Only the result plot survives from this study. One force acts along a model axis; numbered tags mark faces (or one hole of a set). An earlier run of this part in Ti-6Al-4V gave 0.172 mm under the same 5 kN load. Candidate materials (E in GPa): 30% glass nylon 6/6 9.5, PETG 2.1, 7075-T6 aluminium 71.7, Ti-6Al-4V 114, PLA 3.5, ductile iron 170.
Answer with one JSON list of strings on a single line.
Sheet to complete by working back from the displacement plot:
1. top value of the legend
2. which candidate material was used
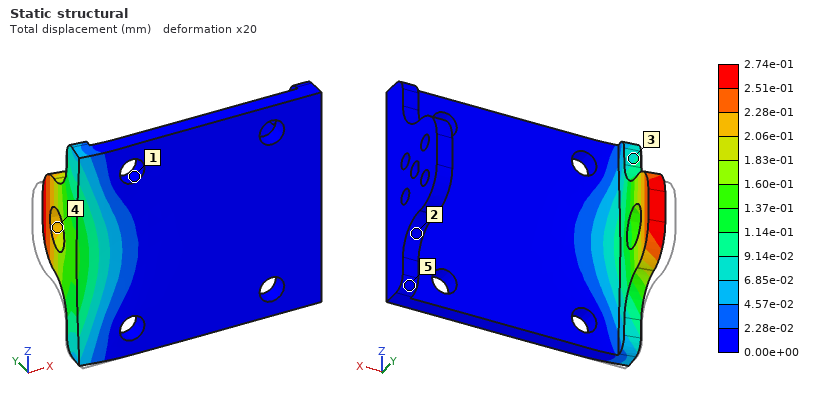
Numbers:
["2.74e-01 mm", "7075-T6 aluminium"]
